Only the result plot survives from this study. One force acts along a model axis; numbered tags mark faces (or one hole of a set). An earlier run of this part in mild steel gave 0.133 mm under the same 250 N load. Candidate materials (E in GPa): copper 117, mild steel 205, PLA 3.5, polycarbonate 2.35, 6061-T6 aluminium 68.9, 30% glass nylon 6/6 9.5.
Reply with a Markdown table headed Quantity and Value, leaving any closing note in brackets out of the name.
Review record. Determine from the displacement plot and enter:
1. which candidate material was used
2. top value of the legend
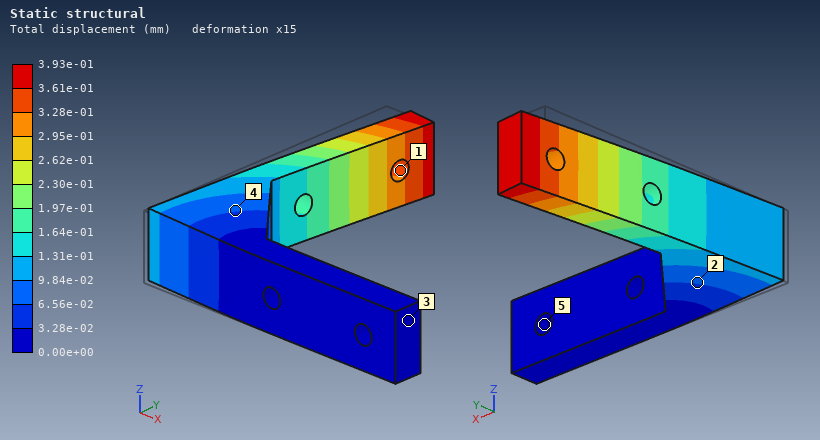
| Quantity | Value |
|---|---|
| which candidate material was used | 6061-T6 aluminium |
| top value of the legend | 3.93e-01 mm |
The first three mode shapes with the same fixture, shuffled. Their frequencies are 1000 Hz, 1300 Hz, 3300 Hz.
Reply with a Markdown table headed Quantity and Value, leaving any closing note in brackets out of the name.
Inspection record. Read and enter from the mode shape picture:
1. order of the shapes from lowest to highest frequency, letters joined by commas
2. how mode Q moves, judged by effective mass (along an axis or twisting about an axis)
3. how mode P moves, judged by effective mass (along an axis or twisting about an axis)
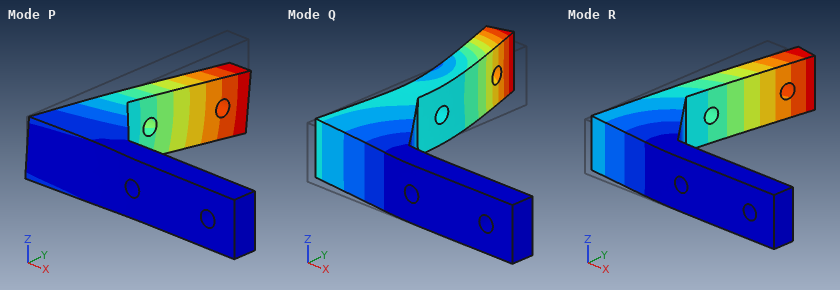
| Quantity | Value |
|---|---|
| order of the shapes from lowest to highest frequency, letters joined by commas | R, P, Q |
| how mode Q moves, judged by effective mass | along Y |
| how mode P moves, judged by effective mass | along Z |
